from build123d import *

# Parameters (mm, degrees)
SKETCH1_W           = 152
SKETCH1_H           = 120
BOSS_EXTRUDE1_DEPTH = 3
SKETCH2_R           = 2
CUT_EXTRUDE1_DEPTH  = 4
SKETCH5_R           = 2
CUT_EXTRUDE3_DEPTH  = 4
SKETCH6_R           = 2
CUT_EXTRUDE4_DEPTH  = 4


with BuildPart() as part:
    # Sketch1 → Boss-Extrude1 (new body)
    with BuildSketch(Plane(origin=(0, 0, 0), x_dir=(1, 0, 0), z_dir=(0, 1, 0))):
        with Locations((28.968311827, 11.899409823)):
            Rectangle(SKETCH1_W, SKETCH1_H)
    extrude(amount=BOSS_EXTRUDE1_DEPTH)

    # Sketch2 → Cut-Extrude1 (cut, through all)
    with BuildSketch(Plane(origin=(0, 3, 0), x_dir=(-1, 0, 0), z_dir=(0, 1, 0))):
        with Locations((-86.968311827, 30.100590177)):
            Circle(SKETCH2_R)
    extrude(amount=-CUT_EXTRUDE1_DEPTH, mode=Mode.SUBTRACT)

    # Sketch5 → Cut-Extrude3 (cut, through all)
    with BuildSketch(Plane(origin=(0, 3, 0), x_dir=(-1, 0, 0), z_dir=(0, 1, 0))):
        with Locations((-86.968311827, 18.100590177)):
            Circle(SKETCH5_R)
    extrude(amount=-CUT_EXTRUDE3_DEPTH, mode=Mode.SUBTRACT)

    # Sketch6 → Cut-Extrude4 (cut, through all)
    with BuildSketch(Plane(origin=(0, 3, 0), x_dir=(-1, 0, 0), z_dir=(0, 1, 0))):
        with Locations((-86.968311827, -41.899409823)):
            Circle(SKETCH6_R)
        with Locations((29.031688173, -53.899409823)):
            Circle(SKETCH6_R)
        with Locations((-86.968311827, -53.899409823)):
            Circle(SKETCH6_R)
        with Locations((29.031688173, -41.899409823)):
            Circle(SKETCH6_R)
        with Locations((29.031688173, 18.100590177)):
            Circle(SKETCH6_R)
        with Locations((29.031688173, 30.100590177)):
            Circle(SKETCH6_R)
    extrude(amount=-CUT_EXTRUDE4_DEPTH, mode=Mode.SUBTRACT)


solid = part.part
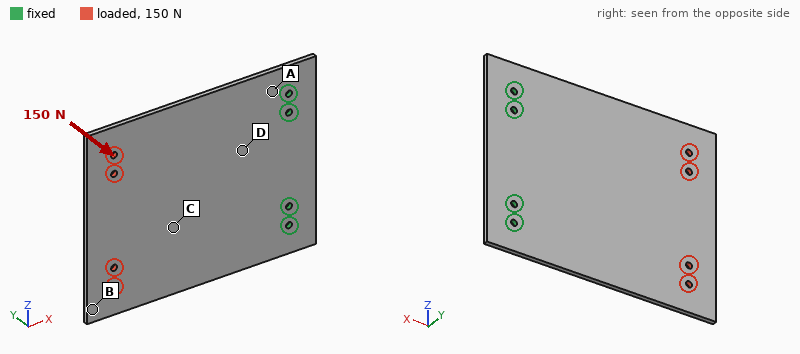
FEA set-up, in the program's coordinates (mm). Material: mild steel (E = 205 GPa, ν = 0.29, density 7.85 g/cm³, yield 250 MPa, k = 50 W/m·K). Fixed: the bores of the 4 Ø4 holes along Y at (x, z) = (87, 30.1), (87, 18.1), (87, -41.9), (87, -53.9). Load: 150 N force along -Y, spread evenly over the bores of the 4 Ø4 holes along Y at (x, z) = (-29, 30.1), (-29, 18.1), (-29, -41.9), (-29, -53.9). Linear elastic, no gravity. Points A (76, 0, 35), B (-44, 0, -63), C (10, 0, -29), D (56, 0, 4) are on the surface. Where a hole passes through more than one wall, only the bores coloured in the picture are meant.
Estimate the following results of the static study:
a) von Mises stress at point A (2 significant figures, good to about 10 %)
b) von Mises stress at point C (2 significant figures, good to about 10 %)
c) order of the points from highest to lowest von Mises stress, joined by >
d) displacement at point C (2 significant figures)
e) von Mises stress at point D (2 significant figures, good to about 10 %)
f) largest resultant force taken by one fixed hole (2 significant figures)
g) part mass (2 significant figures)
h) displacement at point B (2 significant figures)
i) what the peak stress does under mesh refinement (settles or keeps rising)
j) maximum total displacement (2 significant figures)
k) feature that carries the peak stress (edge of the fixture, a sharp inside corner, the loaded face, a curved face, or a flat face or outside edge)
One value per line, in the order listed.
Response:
90 MPa
31 MPa
A > D > C > B
0.76 mm
64 MPa
97 N
430 g
1.7 mm
keeps rising
1.8 mm
edge of the fixture
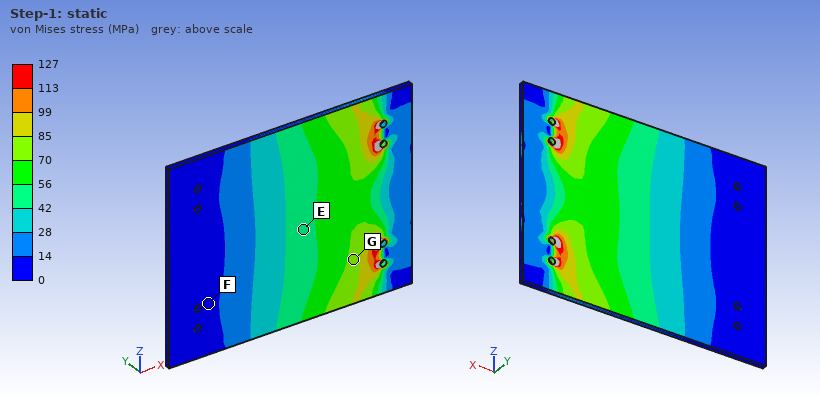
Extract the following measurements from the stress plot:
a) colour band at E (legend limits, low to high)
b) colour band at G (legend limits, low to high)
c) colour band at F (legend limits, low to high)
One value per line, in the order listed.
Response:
42 to 56 MPa
70 to 85 MPa
0 to 14 MPa
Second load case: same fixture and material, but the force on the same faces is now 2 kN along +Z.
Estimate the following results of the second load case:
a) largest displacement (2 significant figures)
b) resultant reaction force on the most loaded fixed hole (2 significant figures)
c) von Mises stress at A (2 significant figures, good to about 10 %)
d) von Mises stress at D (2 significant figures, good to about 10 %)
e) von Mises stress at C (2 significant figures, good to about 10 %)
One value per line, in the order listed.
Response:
32 µm
2.2 kN
27 MPa
17 MPa
14 MPa
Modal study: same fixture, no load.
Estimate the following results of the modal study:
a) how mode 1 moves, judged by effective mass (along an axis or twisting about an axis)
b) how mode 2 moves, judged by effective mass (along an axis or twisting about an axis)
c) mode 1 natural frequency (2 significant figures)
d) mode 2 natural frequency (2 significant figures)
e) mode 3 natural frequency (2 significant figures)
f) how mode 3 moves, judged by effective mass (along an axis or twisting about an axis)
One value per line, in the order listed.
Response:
along Y
twisting about X
140 Hz
370 Hz
840 Hz
along Y
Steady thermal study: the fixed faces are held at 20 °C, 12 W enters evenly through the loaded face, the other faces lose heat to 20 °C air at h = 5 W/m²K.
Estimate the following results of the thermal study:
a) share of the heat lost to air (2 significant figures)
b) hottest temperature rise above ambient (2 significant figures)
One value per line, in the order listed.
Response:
43 %
62 K
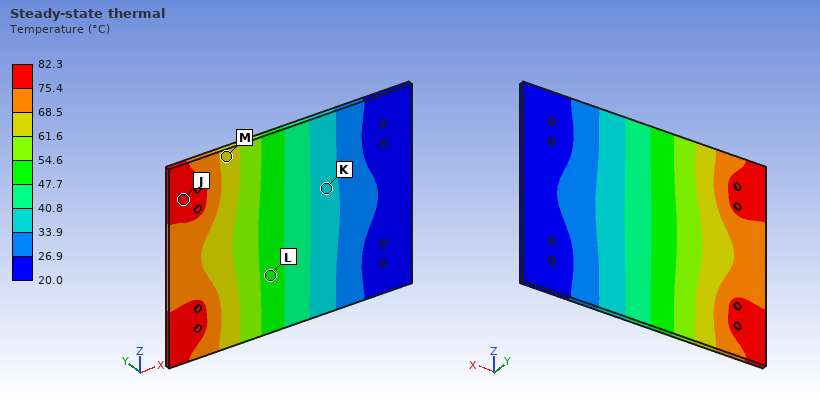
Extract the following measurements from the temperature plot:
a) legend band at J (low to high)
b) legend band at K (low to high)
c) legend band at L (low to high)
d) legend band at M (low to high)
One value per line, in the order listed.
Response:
75.4 to 82.3 °C
33.9 to 40.8 °C
47.7 to 54.6 °C
61.6 to 68.5 °C
